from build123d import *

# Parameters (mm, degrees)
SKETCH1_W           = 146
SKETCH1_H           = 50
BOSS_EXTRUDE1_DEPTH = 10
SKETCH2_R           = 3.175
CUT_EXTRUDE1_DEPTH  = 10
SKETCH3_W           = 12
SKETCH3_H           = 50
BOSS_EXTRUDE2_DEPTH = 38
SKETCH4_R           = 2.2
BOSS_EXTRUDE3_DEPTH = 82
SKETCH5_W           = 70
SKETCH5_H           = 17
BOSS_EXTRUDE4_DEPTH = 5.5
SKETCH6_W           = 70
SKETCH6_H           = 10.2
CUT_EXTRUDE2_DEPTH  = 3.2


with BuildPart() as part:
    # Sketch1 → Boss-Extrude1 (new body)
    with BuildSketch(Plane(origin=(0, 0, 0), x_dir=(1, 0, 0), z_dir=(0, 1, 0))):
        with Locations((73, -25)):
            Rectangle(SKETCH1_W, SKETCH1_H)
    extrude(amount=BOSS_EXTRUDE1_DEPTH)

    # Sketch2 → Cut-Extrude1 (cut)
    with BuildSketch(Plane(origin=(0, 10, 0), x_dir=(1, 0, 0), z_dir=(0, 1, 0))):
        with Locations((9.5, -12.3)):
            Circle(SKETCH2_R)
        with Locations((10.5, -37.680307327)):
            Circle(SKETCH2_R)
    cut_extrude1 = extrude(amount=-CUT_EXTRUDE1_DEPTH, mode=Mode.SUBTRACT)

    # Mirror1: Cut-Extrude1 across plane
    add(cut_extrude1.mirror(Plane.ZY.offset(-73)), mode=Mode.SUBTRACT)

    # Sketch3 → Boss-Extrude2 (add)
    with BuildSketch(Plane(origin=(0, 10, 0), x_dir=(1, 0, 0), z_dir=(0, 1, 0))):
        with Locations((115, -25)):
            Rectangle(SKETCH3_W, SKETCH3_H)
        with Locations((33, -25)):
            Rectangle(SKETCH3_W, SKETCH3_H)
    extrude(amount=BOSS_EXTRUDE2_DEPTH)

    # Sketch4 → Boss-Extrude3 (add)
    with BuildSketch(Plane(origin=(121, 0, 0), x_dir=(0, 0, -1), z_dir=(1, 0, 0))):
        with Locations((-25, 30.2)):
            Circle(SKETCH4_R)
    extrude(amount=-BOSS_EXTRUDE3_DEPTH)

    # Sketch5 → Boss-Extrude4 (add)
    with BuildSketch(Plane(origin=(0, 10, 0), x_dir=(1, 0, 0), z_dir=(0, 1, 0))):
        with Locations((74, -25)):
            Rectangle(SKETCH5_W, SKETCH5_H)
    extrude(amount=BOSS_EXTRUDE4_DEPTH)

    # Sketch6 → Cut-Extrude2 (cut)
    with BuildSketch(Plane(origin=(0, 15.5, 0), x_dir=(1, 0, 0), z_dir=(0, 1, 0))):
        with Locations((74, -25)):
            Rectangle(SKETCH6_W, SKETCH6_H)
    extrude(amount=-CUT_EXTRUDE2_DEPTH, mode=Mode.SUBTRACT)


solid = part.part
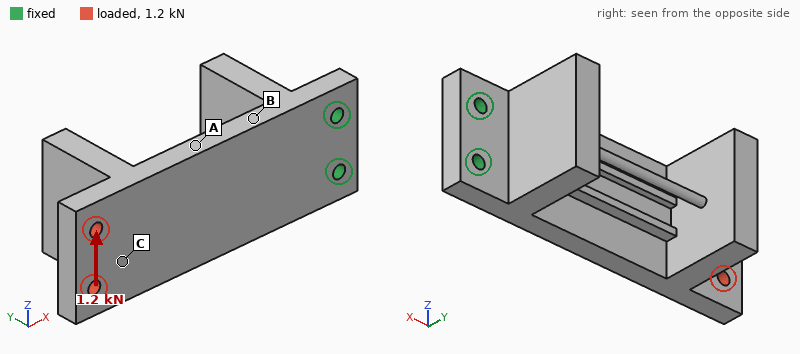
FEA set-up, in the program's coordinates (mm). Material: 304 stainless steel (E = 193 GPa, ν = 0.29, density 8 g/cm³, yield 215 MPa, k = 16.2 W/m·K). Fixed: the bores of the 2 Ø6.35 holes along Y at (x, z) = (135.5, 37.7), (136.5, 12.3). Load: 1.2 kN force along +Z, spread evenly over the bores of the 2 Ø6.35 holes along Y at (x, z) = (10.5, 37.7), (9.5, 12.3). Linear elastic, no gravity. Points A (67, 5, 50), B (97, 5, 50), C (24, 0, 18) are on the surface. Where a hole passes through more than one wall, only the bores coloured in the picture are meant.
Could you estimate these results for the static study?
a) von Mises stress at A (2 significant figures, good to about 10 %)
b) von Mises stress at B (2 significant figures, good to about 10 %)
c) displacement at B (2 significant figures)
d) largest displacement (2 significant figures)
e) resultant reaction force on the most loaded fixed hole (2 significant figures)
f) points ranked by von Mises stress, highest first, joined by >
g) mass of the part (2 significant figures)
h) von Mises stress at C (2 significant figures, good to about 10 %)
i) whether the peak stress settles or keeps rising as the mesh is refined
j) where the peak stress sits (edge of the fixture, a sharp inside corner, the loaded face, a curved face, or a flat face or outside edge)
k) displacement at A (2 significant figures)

16 MPa
24 MPa
11 µm
56 µm
5.1 kN
B > A > C
980 g
6.0 MPa
keeps rising
edge of the fixture
23 µm
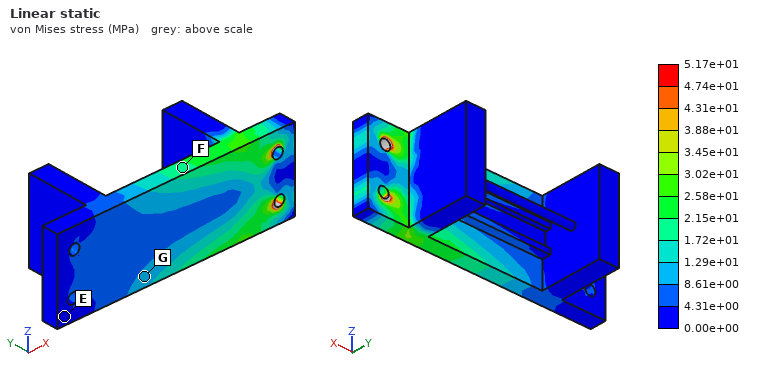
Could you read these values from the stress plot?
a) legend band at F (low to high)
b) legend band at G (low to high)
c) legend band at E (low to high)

1.72e+01 to 2.15e+01 MPa
8.61e+00 to 1.29e+01 MPa
0.00e+00 to 4.31e+00 MPa
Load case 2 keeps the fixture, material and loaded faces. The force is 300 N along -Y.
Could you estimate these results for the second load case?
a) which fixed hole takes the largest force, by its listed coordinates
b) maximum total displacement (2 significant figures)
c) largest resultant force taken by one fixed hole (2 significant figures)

(135.5, 37.7)
0.15 mm
190 N
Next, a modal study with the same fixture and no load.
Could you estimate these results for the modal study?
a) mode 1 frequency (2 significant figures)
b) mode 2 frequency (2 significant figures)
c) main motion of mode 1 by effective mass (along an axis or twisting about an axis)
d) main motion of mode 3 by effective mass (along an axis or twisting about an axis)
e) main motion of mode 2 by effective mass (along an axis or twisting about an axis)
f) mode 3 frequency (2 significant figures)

420 Hz
1200 Hz
along Y
along Z
along Z
1800 Hz
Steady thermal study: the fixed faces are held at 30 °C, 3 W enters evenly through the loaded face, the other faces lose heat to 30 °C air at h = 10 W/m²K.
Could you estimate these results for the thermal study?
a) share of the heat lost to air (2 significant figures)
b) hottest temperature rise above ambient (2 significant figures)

73 %
21 K
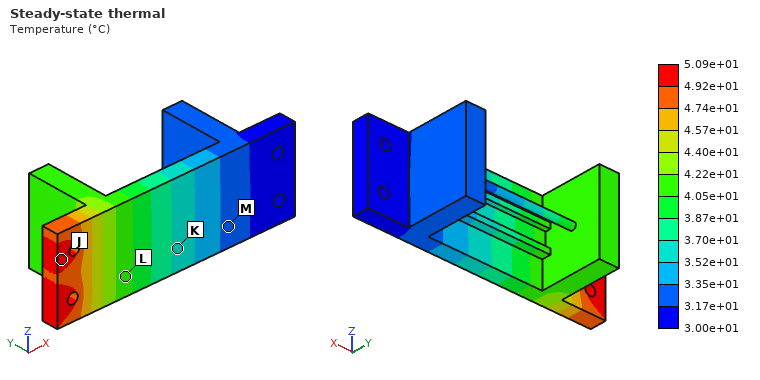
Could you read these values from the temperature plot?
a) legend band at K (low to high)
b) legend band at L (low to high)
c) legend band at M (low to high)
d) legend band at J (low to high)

3.52e+01 to 3.70e+01 °C
4.05e+01 to 4.22e+01 °C
3.17e+01 to 3.35e+01 °C
4.92e+01 to 5.09e+01 °C
